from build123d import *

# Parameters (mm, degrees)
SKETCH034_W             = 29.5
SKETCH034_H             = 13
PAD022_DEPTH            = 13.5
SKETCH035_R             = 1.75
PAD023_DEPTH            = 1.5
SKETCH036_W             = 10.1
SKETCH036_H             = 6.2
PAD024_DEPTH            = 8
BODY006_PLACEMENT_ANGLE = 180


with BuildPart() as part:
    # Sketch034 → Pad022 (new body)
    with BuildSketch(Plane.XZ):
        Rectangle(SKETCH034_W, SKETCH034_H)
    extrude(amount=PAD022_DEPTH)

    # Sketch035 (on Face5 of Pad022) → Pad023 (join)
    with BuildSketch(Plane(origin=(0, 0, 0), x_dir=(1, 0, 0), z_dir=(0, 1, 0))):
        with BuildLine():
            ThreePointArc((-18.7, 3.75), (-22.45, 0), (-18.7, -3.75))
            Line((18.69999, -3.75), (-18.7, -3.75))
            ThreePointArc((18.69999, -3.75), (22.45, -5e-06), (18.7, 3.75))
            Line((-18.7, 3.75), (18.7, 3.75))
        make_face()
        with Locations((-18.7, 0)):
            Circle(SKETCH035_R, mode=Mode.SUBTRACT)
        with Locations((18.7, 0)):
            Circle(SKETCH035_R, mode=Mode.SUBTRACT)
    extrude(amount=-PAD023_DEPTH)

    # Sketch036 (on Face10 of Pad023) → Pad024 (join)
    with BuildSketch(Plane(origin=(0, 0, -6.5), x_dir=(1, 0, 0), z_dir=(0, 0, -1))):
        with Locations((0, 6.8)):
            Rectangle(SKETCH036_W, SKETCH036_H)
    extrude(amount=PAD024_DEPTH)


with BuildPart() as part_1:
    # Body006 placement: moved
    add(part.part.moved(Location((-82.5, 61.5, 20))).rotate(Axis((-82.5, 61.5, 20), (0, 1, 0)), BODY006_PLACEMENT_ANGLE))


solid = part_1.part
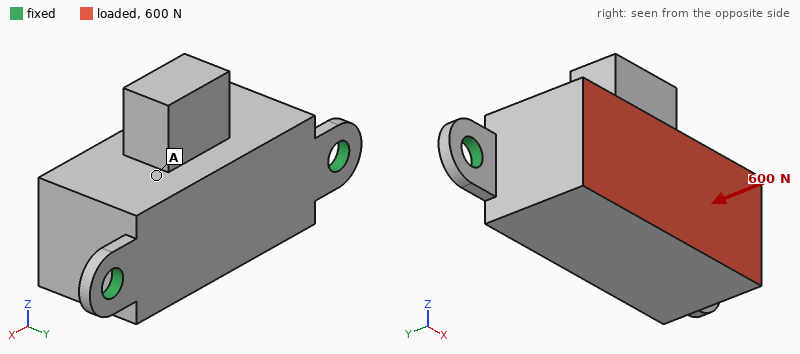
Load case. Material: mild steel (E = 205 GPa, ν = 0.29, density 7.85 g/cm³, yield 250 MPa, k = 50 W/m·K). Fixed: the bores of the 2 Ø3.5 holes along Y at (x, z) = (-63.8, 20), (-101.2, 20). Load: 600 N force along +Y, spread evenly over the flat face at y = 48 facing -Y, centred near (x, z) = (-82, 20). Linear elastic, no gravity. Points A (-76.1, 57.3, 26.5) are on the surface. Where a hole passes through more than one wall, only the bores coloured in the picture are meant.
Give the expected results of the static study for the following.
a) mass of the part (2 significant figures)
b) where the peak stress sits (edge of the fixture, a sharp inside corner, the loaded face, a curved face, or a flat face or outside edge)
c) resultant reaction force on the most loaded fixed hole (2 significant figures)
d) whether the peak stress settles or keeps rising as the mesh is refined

46 g
edge of the fixture
350 N
keeps rising
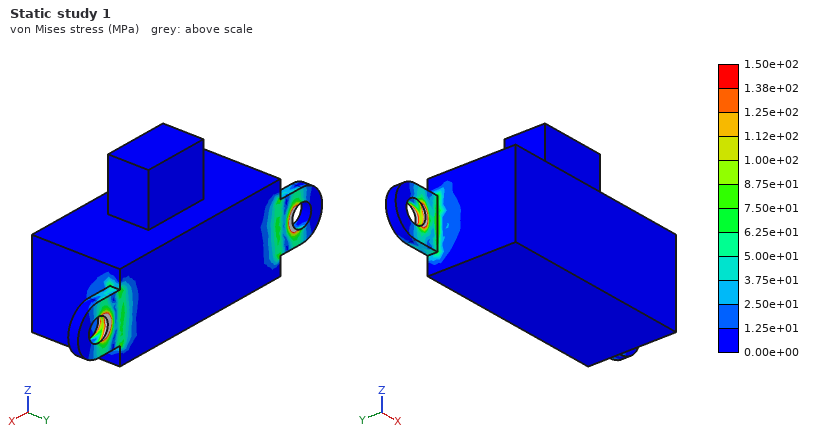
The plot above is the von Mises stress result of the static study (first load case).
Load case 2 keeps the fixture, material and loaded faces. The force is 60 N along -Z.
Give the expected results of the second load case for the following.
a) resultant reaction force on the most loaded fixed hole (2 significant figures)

30 N
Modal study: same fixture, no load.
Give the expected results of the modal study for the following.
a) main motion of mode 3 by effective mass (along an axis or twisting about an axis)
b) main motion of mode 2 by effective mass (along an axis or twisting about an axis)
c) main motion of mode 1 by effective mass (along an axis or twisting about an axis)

along X
along Y
along Z
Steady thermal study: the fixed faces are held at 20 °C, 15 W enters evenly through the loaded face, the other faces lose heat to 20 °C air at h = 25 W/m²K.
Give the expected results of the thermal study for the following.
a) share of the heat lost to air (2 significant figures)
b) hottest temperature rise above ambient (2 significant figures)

16 %
60 K
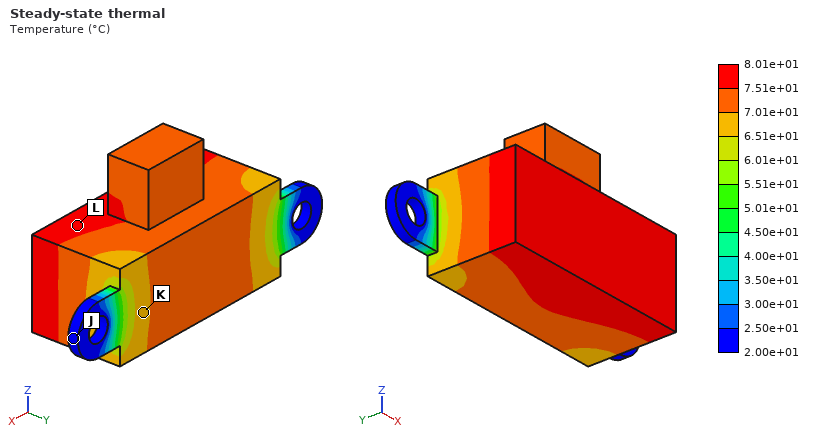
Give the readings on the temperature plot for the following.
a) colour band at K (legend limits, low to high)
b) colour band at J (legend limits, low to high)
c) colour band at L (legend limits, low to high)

6.51e+01 to 7.01e+01 °C
2.00e+01 to 2.50e+01 °C
7.51e+01 to 8.01e+01 °C
